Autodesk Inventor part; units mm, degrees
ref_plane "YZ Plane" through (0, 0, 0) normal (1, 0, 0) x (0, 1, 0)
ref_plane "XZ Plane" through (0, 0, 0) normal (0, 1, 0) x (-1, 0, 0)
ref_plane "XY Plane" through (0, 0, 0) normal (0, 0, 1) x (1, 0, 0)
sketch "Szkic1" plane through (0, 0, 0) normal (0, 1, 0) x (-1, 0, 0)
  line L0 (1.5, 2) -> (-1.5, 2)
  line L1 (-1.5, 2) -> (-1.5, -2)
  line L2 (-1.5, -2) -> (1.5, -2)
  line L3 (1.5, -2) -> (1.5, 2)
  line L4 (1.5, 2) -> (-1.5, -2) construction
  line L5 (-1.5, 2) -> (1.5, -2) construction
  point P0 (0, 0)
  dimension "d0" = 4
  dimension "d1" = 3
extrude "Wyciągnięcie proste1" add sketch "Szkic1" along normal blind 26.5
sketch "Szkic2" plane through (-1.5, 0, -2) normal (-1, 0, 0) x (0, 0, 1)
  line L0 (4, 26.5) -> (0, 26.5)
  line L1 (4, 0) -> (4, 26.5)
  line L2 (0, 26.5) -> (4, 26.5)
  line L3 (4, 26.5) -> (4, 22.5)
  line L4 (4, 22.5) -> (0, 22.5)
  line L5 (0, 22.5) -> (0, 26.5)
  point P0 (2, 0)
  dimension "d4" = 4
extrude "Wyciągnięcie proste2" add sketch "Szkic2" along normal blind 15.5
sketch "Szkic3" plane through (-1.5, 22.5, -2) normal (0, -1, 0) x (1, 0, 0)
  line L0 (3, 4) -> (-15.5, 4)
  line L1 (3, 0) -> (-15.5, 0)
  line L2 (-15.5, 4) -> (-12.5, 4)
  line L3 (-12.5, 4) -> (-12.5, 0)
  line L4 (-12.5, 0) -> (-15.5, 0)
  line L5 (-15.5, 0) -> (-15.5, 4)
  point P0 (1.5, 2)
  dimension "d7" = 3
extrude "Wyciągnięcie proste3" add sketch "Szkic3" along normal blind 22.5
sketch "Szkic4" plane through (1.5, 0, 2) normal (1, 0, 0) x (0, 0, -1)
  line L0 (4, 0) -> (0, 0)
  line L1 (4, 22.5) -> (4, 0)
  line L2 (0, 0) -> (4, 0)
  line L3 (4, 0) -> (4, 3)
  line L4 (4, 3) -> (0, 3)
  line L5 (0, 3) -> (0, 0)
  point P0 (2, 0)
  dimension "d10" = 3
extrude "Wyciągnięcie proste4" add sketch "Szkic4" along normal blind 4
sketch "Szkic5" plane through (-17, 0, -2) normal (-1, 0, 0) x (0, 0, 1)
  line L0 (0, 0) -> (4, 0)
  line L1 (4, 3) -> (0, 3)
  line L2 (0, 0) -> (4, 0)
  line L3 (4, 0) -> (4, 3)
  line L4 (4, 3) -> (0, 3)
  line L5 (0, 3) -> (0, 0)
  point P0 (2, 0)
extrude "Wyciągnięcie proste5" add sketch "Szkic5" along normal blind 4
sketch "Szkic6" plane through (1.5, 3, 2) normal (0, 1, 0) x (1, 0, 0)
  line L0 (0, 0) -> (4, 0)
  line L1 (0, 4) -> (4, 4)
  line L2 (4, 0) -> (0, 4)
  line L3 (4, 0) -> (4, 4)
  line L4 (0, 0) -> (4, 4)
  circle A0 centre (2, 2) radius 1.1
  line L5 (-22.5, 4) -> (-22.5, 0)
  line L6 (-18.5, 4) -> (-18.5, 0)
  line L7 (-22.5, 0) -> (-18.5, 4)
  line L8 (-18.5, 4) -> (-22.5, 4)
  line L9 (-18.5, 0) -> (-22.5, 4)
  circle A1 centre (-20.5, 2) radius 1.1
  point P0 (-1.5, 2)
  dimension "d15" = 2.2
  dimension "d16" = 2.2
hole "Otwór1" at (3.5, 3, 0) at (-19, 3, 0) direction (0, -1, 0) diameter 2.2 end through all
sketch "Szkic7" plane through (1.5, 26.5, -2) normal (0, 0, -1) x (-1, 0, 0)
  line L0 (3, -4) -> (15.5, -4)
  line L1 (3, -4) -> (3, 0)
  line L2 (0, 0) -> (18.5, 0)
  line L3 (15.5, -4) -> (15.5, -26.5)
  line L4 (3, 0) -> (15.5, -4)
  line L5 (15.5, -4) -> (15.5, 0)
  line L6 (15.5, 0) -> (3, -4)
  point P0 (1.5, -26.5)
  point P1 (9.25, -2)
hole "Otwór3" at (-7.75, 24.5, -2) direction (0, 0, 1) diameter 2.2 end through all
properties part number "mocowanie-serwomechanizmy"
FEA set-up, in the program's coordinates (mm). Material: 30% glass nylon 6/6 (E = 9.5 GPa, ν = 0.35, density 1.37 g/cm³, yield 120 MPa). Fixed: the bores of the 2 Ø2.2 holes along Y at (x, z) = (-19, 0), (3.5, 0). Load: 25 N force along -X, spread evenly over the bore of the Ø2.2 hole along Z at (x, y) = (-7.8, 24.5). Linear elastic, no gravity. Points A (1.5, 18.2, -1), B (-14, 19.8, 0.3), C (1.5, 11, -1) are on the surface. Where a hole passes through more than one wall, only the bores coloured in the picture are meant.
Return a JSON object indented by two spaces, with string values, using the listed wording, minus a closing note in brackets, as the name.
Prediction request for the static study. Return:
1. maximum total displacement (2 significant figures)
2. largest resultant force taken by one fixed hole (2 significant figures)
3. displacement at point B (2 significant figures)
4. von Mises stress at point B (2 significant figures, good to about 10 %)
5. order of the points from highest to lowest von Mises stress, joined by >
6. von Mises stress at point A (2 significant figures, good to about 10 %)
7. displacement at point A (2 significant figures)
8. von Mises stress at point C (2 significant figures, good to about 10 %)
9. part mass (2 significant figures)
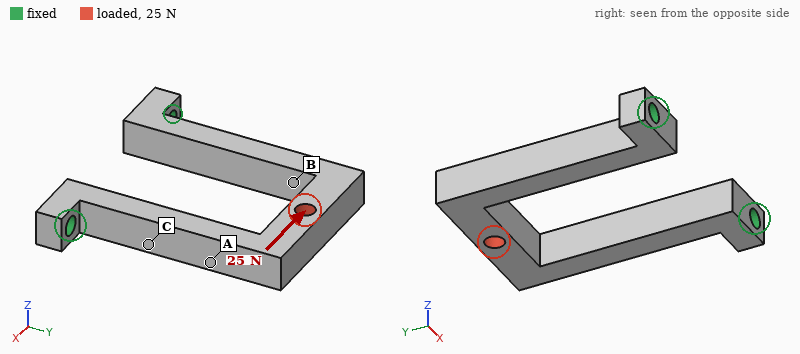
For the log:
{
  "maximum total displacement": "0.18 mm",
  "largest resultant force taken by one fixed hole": "23 N",
  "displacement at point B": "0.16 mm",
  "von Mises stress at point B": "16 MPa",
  "order of the points from highest to lowest von Mises stress, joined by >": "B > A > C",
  "von Mises stress at point A": "10 MPa",
  "displacement at point A": "0.15 mm",
  "von Mises stress at point C": "4.7 MPa",
  "part mass": "1.2 g"
}
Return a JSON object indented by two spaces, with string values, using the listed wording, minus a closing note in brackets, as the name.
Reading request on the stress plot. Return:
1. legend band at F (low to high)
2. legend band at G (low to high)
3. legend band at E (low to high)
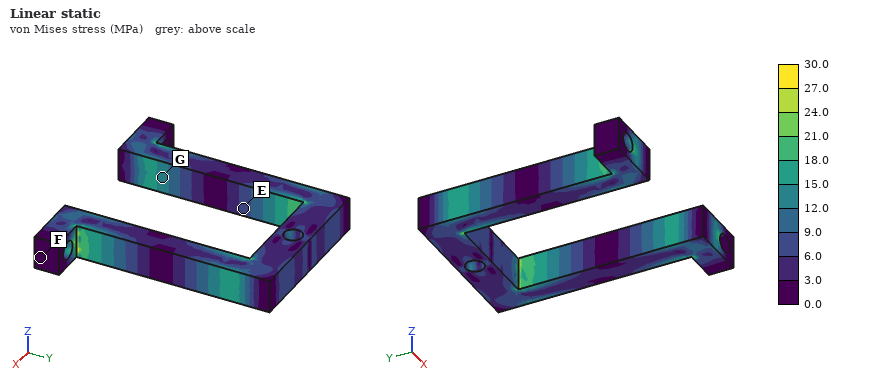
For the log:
{
  "legend band at F": "0.0 to 3.0 MPa",
  "legend band at G": "12.0 to 15.0 MPa",
  "legend band at E": "6.0 to 9.0 MPa"
}
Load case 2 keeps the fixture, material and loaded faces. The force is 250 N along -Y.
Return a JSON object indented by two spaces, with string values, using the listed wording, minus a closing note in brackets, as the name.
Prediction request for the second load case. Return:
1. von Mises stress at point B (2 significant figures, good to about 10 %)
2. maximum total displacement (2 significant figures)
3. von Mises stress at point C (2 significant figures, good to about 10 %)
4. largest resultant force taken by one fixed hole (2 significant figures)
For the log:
{
  "von Mises stress at point B": "35 MPa",
  "maximum total displacement": "0.11 mm",
  "von Mises stress at point C": "9.6 MPa",
  "largest resultant force taken by one fixed hole": "130 N"
}
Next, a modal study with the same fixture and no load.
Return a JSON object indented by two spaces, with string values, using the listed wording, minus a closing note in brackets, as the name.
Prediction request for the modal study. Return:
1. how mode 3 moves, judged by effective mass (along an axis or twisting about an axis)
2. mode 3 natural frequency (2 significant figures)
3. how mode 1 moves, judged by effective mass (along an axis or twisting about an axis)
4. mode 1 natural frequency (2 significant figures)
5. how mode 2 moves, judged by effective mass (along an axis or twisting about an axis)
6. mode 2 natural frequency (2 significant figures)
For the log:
{
  "how mode 3 moves, judged by effective mass": "twisting about Y",
  "mode 3 natural frequency": "3700 Hz",
  "how mode 1 moves, judged by effective mass": "along Z",
  "mode 1 natural frequency": "1500 Hz",
  "how mode 2 moves, judged by effective mass": "along X",
  "mode 2 natural frequency": "2400 Hz"
}
